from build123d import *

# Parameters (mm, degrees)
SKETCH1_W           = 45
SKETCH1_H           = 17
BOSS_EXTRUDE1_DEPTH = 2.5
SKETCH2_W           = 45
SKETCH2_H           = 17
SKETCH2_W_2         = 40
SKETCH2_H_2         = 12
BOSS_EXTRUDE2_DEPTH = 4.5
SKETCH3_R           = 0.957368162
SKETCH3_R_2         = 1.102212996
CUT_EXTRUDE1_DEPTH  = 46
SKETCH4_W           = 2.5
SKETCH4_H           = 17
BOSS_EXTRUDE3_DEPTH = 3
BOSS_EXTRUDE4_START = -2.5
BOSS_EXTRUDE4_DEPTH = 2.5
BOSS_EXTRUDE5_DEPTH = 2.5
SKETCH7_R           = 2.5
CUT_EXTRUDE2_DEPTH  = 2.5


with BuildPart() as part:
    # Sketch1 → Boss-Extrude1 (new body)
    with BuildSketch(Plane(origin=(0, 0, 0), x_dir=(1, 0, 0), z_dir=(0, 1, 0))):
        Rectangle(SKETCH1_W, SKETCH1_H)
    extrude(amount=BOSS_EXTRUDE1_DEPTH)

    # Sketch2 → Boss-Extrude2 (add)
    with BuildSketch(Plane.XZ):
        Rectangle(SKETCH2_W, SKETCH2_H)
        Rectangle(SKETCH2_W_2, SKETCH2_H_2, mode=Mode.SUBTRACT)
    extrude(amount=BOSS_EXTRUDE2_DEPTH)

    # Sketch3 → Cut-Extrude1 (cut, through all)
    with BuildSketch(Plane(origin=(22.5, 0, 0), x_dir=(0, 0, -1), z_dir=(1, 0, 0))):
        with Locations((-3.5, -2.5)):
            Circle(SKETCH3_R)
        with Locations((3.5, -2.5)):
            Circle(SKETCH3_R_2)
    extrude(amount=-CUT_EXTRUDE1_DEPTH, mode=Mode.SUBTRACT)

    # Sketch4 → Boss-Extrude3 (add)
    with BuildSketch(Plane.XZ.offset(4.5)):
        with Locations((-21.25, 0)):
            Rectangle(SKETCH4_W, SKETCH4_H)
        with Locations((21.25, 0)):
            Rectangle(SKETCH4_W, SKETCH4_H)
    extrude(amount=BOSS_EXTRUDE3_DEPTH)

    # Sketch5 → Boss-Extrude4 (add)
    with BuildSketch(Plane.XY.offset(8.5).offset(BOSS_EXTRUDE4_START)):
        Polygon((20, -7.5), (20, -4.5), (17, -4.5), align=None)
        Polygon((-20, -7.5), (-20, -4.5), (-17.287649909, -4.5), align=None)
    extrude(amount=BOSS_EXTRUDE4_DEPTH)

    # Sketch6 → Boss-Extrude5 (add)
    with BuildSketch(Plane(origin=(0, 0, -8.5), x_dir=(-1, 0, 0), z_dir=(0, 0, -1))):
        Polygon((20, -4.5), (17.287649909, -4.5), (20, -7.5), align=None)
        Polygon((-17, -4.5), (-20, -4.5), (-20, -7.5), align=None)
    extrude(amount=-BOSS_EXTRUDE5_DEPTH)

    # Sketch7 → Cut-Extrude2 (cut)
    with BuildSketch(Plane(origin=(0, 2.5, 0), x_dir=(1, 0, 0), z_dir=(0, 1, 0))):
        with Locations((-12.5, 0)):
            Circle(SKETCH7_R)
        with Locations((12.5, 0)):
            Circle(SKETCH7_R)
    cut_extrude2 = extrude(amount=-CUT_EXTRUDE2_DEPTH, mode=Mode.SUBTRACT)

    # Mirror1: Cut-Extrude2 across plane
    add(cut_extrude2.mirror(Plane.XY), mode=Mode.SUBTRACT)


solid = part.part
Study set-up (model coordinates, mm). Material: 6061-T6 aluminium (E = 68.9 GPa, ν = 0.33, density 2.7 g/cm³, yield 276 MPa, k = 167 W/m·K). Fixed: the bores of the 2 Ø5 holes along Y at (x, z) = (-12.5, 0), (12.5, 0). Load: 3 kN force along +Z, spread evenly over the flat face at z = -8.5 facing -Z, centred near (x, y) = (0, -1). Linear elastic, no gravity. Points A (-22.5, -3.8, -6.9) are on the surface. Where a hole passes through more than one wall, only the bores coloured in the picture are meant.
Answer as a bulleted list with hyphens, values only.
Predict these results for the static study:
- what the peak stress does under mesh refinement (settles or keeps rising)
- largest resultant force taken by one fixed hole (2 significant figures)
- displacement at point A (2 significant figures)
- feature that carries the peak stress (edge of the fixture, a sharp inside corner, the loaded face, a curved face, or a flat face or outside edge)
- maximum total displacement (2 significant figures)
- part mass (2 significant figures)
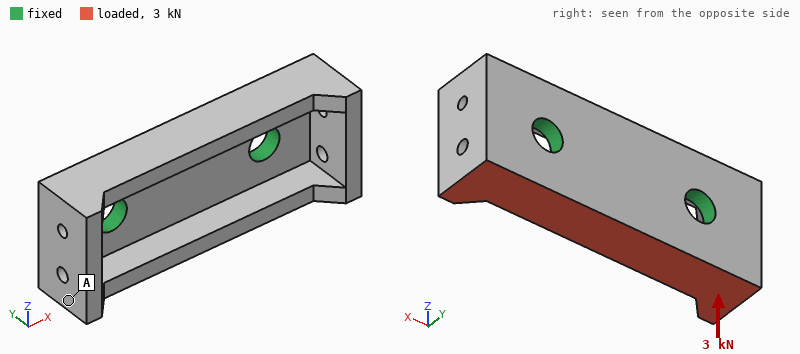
- keeps rising
- 1.5 kN
- 37 µm
- edge of the fixture
- 71 µm
- 9.1 g
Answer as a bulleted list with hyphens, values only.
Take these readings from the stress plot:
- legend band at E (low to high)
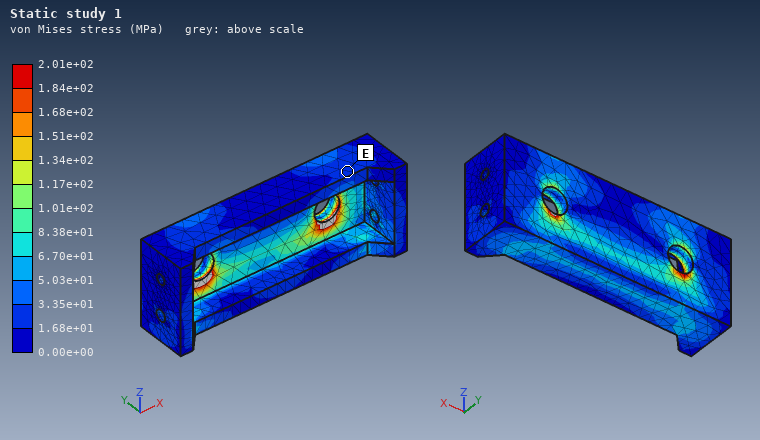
- 1.68e+01 to 3.35e+01 MPa
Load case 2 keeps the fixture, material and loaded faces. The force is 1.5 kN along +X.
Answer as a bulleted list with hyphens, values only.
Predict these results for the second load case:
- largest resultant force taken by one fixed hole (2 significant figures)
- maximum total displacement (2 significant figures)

- 850 N
- 20 µm
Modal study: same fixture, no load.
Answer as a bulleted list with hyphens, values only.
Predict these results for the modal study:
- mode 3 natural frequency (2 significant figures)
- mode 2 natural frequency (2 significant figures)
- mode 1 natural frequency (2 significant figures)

- 18 kHz
- 14 kHz
- 14 kHz
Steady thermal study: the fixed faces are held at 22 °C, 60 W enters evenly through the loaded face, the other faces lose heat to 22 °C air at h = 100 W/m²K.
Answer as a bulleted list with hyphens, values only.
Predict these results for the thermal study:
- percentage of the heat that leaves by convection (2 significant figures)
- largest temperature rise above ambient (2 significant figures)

- 5.5 %
- 30 K
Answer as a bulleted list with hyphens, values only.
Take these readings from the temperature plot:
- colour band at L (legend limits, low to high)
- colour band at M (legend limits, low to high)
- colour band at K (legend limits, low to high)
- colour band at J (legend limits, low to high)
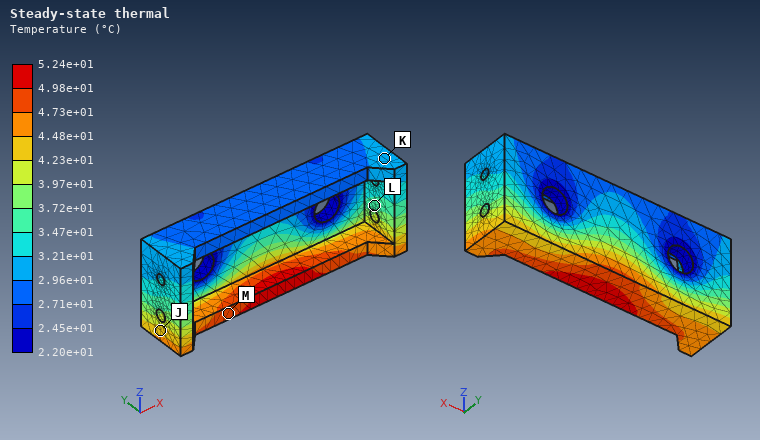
- 3.47e+01 to 3.72e+01 °C
- 4.73e+01 to 4.98e+01 °C
- 2.96e+01 to 3.21e+01 °C
- 4.23e+01 to 4.48e+01 °C
